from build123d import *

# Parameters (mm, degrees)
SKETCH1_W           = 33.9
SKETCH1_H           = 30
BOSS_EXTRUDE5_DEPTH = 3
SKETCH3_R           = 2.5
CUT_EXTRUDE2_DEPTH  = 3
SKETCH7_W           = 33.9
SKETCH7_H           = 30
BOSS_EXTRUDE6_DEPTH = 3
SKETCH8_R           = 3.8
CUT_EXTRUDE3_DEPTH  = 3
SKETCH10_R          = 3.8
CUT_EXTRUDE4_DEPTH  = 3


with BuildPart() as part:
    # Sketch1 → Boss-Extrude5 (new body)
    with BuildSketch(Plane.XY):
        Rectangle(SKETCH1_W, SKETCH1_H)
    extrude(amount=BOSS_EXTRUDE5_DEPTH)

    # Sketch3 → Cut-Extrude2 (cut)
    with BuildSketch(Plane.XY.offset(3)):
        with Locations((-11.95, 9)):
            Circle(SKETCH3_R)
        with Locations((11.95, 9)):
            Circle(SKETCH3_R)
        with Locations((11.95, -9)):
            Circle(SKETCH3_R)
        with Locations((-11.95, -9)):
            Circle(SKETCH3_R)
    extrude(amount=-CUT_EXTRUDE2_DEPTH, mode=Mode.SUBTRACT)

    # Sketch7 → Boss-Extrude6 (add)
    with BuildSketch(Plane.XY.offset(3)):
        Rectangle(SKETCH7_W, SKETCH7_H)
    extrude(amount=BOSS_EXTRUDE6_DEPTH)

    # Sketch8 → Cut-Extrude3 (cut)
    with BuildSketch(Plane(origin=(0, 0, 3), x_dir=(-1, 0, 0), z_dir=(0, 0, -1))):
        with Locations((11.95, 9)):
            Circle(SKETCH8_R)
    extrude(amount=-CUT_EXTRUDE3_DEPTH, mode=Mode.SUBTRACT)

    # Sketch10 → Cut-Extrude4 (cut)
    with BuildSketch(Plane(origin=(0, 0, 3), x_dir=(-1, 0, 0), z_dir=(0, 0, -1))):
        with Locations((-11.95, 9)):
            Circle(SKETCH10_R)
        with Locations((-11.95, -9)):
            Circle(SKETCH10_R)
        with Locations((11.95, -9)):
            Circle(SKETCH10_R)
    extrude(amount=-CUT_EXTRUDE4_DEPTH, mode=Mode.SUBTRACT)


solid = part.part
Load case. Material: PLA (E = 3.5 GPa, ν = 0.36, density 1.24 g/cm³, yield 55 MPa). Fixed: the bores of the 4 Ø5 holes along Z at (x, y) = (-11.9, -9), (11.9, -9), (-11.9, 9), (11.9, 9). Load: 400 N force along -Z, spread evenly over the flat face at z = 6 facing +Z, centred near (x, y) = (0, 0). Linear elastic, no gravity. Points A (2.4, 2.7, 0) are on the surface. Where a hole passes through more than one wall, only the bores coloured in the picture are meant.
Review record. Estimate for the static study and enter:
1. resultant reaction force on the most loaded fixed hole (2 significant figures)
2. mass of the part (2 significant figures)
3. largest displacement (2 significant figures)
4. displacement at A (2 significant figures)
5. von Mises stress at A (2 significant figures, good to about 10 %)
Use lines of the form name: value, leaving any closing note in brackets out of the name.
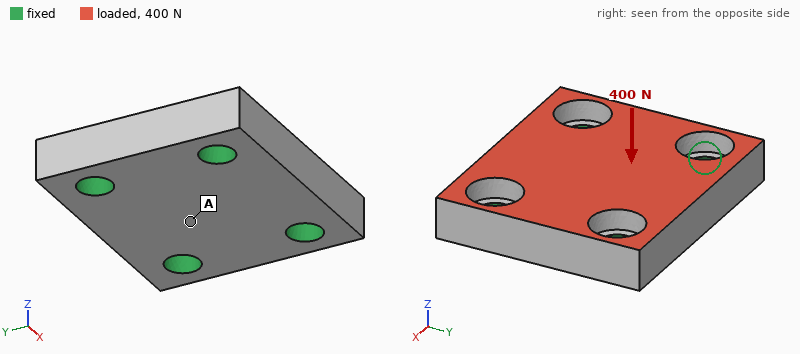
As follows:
resultant reaction force on the most loaded fixed hole: 110 N
mass of the part: 6.6 g
largest displacement: 15 µm
displacement at A: 14 µm
von Mises stress at A: 1.5 MPa
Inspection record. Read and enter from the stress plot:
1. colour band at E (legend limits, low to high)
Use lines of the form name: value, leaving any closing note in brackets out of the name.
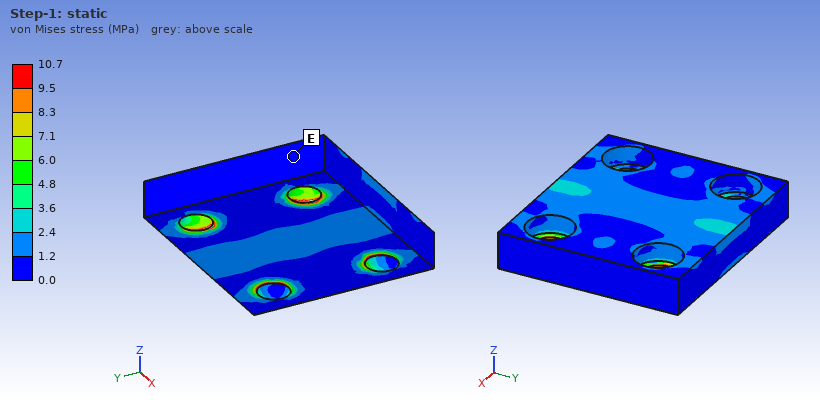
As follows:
colour band at E: 0.0 to 1.2 MPa
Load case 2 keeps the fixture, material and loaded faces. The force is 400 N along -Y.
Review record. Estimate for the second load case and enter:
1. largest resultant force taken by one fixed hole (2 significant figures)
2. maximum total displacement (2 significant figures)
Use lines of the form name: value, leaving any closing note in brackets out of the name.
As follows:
largest resultant force taken by one fixed hole: 110 N
maximum total displacement: 18 µm
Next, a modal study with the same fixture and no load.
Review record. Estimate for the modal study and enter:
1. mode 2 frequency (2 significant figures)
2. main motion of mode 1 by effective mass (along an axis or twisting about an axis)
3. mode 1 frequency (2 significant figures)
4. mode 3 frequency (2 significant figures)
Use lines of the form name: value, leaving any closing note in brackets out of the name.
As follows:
mode 2 frequency: 13 kHz
main motion of mode 1 by effective mass: along Z
mode 1 frequency: 11 kHz
mode 3 frequency: 16 kHz
